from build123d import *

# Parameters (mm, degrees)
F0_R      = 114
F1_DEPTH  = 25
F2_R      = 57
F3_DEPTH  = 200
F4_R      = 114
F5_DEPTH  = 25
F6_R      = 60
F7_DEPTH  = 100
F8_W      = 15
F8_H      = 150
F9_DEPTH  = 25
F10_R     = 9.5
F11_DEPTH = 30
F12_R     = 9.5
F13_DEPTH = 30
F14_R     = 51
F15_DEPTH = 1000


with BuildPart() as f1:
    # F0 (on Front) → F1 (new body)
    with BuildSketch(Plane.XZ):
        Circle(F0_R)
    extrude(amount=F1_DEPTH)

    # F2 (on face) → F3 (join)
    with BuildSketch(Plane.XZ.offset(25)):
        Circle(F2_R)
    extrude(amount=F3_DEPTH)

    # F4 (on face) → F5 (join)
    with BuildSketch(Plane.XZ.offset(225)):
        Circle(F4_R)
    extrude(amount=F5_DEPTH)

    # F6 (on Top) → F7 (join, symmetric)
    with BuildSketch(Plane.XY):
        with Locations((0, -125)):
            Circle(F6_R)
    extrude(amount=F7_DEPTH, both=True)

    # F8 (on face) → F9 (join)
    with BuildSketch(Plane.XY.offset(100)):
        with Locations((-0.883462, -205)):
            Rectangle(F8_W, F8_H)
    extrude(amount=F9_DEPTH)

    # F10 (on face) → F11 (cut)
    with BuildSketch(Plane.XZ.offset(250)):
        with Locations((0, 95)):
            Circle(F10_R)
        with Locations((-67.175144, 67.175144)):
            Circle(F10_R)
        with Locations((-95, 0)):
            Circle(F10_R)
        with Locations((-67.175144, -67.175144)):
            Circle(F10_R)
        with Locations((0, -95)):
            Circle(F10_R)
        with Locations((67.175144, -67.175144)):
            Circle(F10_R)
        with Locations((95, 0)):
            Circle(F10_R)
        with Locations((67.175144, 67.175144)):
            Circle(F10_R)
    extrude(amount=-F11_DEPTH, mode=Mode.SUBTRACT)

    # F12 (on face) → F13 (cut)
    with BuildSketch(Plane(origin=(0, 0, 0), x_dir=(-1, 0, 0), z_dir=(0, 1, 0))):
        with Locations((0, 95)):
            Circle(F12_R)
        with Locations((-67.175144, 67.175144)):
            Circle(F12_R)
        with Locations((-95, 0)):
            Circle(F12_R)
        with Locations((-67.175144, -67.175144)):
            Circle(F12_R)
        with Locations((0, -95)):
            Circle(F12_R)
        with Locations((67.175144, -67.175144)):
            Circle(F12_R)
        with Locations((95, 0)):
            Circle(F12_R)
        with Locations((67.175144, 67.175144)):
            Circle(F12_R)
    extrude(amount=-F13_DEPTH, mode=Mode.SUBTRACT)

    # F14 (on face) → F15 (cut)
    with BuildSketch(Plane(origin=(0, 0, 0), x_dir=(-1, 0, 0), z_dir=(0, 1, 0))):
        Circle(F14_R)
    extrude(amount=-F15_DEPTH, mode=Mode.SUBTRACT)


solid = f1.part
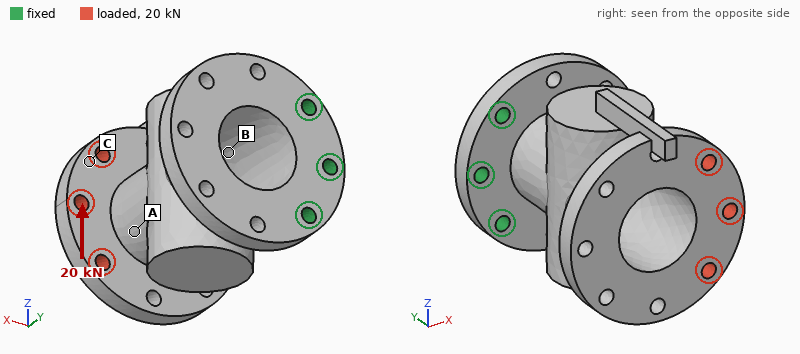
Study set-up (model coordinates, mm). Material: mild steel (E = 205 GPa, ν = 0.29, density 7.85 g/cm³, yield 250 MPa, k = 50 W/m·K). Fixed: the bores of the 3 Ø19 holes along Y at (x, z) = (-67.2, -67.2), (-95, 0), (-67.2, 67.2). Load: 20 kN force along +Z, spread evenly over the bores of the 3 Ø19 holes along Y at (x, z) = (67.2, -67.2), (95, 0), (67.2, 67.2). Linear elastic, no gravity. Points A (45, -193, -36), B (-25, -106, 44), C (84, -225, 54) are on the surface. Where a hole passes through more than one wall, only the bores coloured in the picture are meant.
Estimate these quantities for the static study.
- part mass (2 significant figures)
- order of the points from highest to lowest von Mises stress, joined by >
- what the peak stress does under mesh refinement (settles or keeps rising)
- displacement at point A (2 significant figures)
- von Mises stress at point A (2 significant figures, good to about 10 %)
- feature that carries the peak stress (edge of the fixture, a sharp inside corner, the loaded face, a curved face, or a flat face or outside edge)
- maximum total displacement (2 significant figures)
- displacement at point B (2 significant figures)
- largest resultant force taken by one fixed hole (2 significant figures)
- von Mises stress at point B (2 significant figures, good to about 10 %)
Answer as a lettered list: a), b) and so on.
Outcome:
a) 25 kg
b) A > B > C
c) keeps rising
d) 0.34 mm
e) 45 MPa
f) edge of the fixture
g) 0.52 mm
h) 0.16 mm
i) 43 kN
j) 26 MPa
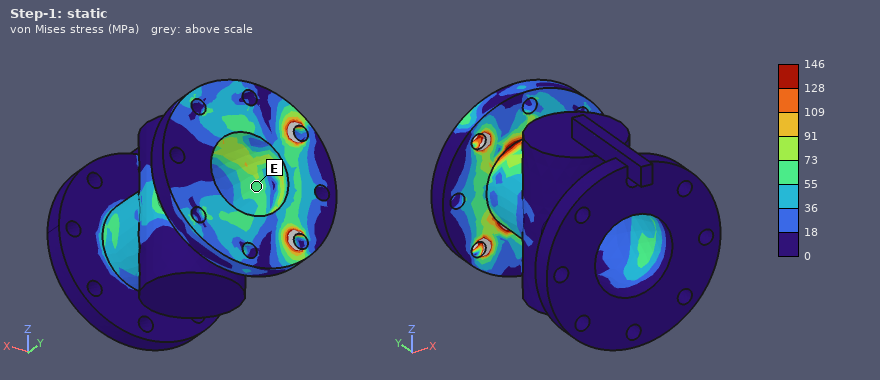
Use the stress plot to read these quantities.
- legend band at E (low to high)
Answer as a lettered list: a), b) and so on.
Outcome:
a) 55 to 73 MPa
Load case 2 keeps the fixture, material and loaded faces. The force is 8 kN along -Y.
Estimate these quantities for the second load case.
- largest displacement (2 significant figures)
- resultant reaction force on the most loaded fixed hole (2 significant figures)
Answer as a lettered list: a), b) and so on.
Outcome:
a) 0.40 mm
b) 7.6 kN
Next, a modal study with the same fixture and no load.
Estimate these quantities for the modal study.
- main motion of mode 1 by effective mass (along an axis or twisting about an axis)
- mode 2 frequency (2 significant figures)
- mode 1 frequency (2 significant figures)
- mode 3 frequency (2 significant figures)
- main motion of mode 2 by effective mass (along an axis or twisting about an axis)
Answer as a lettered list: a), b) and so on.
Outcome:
a) along X
b) 340 Hz
c) 180 Hz
d) 900 Hz
e) along Z
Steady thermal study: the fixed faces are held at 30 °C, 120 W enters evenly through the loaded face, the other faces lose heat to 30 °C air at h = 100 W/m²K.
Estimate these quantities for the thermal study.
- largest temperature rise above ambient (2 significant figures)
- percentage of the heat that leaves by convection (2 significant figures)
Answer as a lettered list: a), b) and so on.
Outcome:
a) 33 K
b) 100 %
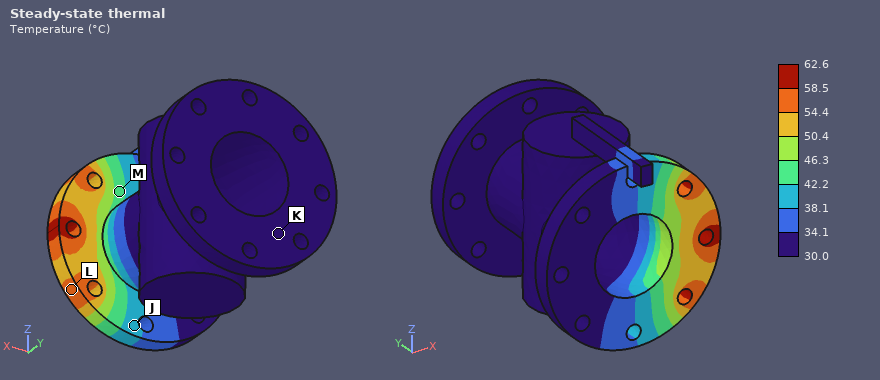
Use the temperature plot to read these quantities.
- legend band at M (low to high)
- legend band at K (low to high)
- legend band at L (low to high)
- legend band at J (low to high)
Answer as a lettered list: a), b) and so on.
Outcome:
a) 42.2 to 46.3 °C
b) 30.0 to 34.1 °C
c) 54.4 to 58.5 °C
d) 38.1 to 42.2 °C
